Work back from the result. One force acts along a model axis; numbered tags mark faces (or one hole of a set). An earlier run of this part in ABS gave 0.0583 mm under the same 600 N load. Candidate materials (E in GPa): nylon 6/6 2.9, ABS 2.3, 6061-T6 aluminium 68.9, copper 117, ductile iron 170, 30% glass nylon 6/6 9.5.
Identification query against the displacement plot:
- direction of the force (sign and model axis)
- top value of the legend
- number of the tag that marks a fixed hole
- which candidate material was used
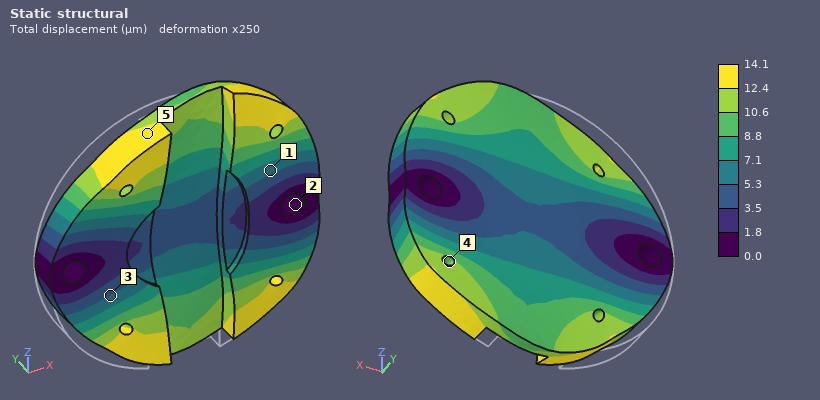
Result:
+X
14.1 µm
2
30% glass nylon 6/6
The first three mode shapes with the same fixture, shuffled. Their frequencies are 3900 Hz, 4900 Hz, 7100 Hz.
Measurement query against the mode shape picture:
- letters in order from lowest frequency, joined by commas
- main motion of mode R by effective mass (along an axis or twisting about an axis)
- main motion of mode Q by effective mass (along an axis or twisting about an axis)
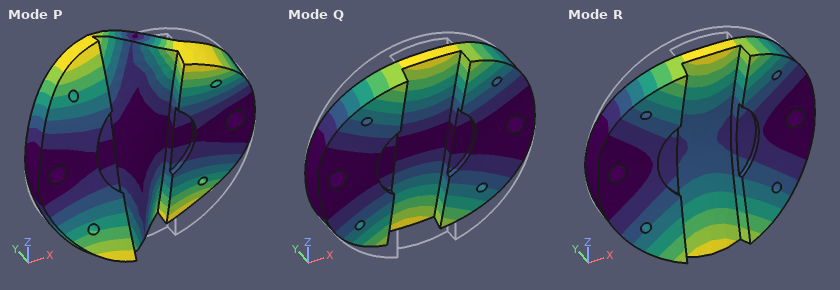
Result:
Q, R, P
along Y
twisting about X
